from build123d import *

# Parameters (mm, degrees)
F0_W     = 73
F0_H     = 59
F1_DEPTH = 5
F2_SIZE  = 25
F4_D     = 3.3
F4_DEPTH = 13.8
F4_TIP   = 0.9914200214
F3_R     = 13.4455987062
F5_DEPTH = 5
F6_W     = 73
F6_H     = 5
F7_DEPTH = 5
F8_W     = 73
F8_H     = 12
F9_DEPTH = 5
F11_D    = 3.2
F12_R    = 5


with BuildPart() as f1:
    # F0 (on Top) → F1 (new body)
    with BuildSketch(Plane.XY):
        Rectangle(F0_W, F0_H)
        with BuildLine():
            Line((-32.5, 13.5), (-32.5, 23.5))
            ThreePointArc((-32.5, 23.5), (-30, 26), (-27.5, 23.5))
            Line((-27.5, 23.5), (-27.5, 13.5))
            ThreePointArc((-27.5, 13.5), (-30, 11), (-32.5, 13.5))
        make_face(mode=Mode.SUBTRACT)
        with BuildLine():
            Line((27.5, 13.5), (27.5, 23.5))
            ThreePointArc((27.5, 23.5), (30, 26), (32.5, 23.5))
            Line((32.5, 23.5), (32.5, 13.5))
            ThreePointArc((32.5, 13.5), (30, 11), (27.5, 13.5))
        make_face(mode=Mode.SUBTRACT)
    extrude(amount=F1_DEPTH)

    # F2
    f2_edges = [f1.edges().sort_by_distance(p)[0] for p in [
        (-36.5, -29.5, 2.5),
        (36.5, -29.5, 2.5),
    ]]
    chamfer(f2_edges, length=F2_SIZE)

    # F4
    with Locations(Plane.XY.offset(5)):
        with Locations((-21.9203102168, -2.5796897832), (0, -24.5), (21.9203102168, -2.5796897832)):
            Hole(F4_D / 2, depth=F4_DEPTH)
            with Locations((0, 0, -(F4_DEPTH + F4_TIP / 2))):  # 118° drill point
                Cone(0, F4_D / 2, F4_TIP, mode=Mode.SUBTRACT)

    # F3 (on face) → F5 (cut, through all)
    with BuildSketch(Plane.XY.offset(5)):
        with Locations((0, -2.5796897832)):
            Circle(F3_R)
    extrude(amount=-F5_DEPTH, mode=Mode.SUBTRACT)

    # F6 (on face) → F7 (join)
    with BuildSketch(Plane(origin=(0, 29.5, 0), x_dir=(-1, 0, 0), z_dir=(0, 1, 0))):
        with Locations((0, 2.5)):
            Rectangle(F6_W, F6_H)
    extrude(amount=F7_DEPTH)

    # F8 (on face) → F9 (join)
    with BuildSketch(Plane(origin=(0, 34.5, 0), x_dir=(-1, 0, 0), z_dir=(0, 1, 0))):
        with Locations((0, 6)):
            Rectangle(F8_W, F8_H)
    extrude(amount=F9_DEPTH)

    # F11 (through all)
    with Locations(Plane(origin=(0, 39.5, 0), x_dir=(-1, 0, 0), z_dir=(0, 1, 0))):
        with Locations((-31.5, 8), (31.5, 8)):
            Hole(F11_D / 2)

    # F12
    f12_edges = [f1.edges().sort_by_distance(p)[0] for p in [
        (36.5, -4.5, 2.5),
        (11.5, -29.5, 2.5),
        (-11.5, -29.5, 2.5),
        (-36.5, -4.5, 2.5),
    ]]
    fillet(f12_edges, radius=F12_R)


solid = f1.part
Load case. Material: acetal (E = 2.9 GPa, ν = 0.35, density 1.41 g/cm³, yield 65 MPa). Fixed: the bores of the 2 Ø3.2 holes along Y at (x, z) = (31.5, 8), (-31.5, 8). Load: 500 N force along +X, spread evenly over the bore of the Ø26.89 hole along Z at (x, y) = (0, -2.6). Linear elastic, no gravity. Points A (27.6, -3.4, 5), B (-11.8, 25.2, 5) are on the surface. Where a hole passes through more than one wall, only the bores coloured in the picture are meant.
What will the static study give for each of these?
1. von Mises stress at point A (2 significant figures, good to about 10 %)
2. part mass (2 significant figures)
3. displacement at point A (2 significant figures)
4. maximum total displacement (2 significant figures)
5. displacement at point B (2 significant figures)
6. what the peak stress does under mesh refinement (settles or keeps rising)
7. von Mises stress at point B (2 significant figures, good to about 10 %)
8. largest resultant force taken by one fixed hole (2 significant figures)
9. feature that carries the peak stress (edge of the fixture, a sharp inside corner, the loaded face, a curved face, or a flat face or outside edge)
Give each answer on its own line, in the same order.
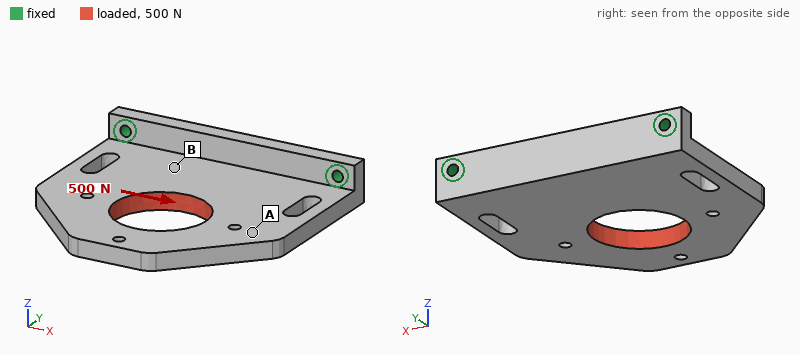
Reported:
3.0 MPa
29 g
0.28 mm
0.34 mm
0.077 mm
keeps rising
4.6 MPa
400 N
edge of the fixture
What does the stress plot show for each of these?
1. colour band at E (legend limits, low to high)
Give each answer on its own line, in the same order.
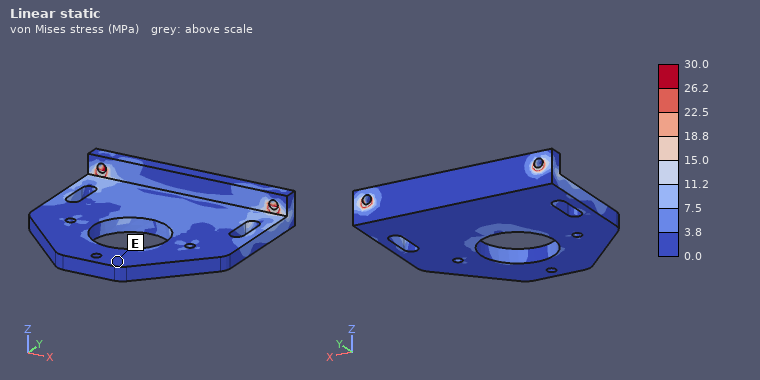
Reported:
0.0 to 3.8 MPa
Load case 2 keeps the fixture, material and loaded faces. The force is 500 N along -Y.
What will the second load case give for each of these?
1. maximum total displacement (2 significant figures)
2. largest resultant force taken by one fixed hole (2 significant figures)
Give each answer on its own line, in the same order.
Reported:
0.79 mm
260 N
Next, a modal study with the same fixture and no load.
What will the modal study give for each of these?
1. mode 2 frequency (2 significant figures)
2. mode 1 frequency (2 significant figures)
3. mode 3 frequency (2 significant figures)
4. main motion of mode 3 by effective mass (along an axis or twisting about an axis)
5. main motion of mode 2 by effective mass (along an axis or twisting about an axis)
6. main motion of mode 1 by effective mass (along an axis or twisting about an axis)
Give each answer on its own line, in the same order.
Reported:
700 Hz
240 Hz
1200 Hz
along Z
twisting about Y
along Z
